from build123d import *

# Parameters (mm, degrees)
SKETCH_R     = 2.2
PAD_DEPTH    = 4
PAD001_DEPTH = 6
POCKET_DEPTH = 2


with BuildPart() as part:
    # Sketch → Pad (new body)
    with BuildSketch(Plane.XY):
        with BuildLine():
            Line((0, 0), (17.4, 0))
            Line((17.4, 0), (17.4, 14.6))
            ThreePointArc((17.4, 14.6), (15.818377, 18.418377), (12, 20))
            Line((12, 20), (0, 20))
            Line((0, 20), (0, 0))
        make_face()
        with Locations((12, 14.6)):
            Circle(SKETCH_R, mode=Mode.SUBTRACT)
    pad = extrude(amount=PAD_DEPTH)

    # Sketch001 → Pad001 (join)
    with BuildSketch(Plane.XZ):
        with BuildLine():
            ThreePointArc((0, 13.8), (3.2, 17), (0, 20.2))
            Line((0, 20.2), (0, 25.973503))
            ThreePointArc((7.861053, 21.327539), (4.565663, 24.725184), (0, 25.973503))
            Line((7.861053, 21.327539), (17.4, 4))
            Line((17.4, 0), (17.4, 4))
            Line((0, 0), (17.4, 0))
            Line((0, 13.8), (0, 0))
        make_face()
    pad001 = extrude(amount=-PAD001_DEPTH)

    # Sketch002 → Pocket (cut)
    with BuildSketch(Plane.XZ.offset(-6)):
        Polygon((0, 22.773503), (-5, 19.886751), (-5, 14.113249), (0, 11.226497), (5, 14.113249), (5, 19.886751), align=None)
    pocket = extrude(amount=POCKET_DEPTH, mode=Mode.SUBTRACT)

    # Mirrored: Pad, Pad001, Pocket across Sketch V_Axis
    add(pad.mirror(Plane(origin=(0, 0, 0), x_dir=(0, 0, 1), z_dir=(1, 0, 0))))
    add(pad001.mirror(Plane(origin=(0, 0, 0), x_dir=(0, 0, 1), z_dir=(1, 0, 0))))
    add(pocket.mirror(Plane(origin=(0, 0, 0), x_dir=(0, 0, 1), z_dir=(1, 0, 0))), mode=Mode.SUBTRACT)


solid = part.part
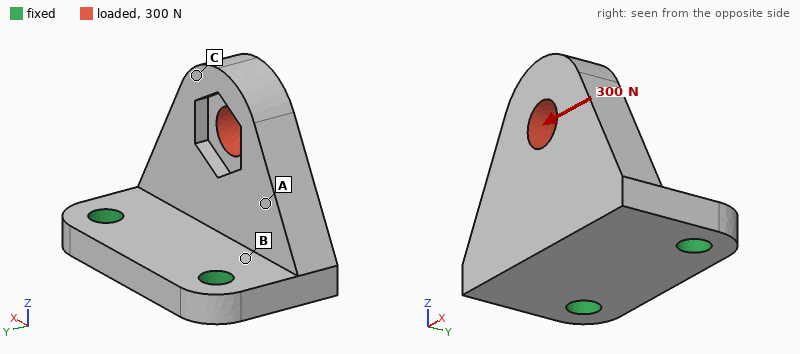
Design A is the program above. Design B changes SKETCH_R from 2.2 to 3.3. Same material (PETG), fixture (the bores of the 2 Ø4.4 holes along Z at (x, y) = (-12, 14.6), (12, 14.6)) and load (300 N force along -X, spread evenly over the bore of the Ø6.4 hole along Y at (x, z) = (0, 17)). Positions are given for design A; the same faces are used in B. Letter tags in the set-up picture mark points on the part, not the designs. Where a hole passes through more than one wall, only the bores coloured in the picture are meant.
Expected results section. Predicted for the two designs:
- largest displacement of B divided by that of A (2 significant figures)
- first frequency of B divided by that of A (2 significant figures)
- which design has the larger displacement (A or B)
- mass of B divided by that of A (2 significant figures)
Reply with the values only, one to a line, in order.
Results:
0.78
1.1
A
0.97
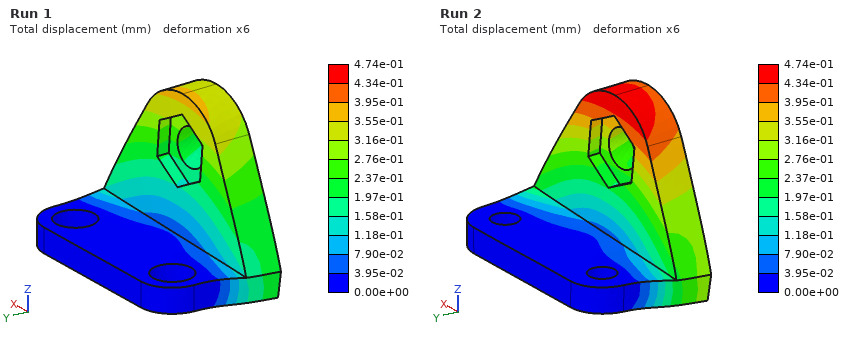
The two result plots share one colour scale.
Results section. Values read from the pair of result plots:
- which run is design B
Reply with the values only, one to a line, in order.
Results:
Run 1
